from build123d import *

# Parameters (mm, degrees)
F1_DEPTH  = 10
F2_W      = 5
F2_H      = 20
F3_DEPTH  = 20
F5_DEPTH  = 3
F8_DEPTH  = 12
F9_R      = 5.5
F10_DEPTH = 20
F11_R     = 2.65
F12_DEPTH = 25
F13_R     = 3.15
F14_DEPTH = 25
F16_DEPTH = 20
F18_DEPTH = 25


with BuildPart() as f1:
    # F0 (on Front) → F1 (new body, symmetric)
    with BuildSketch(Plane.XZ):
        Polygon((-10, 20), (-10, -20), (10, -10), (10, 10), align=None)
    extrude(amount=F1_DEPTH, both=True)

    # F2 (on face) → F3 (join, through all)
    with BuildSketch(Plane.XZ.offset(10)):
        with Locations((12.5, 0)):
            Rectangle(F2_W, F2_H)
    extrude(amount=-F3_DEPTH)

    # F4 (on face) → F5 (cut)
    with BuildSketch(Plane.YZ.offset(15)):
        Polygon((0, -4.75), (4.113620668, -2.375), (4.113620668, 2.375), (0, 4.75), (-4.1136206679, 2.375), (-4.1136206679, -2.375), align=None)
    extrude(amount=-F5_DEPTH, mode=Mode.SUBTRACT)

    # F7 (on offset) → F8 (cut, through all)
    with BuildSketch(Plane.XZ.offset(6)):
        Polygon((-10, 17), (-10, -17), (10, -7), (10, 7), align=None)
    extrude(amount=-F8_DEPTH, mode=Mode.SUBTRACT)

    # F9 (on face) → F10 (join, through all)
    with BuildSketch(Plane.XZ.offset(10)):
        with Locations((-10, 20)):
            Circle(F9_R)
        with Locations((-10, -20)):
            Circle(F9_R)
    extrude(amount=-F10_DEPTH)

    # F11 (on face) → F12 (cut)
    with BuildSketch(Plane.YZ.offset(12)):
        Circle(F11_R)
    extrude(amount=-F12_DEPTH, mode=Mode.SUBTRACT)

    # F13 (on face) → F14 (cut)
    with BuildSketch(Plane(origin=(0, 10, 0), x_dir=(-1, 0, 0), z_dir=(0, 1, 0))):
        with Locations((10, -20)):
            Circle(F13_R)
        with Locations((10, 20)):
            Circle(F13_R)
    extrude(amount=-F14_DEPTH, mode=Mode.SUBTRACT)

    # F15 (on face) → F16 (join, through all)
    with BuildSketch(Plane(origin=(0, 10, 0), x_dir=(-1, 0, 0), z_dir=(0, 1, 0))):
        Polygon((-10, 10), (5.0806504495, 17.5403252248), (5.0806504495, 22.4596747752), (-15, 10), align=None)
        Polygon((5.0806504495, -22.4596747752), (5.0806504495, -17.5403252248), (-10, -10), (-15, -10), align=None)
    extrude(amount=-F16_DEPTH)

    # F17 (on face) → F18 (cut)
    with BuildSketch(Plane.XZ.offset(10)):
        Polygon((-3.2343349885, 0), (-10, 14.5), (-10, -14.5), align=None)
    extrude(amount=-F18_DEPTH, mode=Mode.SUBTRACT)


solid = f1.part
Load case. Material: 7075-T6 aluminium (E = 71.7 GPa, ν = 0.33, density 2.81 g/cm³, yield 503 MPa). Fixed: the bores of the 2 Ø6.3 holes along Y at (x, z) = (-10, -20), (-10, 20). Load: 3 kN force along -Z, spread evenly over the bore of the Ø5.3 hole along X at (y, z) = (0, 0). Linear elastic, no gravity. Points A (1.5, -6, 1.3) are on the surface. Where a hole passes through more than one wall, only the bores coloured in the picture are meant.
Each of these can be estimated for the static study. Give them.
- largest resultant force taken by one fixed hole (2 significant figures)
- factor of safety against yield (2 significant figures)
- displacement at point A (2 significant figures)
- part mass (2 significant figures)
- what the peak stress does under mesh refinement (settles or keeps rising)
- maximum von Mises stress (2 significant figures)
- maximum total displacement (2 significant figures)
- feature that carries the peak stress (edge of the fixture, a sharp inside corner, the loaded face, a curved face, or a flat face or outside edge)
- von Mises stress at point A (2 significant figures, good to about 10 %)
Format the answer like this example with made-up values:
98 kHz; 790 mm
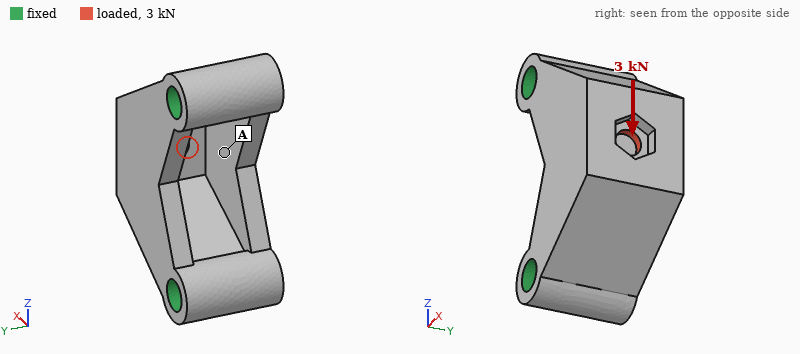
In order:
2.0 kN; 3.2; 4.0 µm; 33 g; settles; 160 MPa; 14 µm; the loaded face; 18 MPa
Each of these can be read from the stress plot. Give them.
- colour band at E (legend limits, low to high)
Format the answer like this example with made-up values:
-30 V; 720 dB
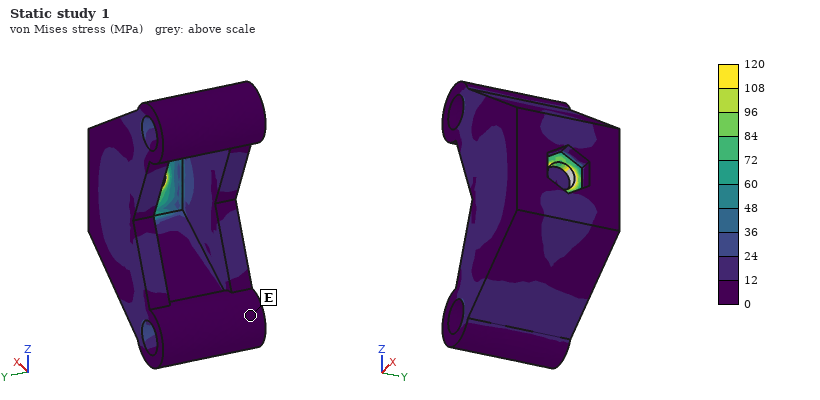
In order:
0 to 12 MPa
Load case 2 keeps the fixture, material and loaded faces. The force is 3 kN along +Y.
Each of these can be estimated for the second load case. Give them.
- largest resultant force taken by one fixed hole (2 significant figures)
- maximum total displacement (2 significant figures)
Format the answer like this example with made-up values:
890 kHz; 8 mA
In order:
1.5 kN; 30 µm
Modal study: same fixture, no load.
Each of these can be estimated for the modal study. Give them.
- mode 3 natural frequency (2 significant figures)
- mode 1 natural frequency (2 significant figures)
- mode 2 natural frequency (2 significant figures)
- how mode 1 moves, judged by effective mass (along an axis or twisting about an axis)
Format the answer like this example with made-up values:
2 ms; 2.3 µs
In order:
28 kHz; 16 kHz; 27 kHz; along Y
